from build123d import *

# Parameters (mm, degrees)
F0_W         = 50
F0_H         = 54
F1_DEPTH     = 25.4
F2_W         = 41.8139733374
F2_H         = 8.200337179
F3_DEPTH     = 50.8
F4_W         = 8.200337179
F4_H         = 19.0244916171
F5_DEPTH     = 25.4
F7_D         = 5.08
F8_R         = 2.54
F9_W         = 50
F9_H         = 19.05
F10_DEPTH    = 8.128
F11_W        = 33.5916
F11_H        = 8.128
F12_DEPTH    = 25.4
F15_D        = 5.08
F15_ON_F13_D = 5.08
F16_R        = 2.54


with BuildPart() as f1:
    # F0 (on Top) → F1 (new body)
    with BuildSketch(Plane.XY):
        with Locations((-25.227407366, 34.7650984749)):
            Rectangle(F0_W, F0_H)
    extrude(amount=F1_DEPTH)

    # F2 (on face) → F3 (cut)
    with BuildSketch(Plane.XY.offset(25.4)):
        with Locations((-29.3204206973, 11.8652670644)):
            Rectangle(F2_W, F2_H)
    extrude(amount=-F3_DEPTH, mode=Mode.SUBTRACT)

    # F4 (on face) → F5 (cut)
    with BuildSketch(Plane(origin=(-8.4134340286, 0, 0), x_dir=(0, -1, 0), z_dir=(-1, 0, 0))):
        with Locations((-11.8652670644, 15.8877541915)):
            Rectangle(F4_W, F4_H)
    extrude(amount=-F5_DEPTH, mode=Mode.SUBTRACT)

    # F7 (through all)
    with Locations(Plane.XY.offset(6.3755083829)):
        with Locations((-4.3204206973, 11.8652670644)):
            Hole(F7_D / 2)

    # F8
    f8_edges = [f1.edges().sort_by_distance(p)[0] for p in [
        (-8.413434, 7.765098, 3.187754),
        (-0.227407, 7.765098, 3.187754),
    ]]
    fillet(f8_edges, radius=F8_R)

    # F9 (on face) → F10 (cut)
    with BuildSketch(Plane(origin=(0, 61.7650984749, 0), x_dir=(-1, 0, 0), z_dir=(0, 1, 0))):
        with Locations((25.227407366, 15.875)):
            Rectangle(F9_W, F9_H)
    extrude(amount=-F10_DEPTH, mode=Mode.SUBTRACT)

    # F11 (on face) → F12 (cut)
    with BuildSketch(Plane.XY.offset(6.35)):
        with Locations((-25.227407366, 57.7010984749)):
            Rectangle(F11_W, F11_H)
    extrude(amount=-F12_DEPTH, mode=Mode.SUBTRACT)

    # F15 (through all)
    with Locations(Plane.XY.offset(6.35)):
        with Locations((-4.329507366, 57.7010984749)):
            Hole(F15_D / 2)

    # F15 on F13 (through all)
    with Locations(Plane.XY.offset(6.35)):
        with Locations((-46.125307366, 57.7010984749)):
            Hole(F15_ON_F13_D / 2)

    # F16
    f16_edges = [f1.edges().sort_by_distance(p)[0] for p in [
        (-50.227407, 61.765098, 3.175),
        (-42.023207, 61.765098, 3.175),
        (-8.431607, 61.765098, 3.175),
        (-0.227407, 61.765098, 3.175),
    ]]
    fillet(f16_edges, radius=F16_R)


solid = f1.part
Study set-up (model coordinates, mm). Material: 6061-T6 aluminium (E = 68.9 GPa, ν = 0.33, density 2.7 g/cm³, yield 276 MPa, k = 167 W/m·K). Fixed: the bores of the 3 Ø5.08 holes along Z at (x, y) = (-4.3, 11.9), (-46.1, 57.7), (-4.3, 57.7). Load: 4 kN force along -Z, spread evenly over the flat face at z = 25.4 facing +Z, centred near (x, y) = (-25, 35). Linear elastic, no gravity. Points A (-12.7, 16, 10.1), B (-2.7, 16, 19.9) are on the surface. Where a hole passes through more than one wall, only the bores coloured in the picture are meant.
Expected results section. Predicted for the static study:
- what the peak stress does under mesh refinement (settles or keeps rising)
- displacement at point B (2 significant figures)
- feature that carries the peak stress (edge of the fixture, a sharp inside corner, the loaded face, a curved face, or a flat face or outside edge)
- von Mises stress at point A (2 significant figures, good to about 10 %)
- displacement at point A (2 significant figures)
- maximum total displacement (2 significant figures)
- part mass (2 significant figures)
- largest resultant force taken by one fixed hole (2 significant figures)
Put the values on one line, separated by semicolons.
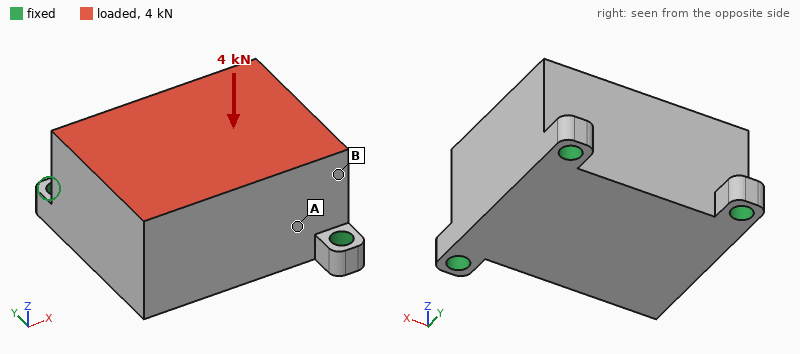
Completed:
keeps rising; 12 µm; edge of the fixture; 19 MPa; 15 µm; 39 µm; 130 g; 2.1 kN
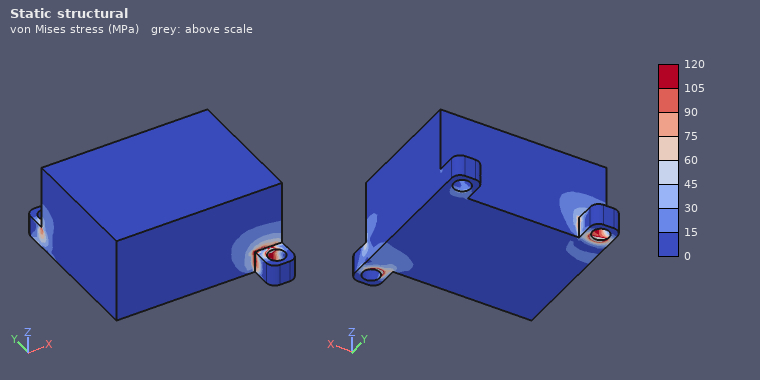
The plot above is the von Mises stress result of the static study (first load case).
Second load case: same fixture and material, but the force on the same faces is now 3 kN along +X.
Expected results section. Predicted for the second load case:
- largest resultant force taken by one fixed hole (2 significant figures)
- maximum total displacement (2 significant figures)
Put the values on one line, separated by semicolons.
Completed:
2.1 kN; 34 µm
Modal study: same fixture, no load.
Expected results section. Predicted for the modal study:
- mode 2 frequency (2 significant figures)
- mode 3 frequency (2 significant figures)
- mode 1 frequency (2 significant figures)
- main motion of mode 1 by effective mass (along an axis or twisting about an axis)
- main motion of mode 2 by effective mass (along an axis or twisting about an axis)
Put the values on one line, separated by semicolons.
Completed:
9400 Hz; 12 kHz; 5400 Hz; along Z; along X
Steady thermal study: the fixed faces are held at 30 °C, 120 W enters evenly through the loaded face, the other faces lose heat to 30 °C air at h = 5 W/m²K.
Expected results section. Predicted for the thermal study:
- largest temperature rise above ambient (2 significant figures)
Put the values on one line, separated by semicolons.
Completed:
41 K
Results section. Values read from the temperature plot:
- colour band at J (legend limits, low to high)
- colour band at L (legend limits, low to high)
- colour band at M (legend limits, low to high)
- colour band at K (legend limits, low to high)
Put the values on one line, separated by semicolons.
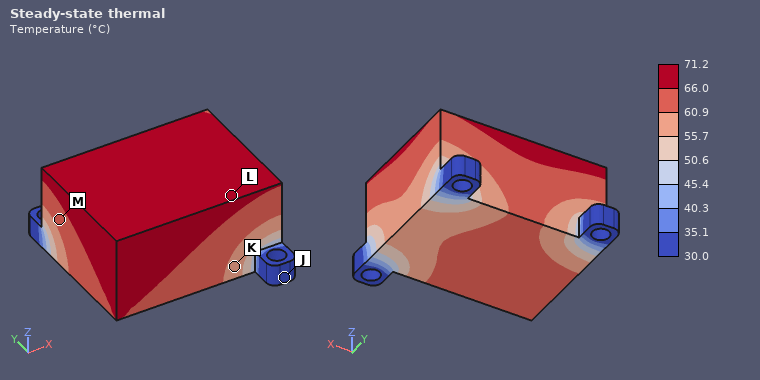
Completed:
30.0 to 35.1 °C; 66.0 to 71.2 °C; 60.9 to 66.0 °C; 55.7 to 60.9 °C
